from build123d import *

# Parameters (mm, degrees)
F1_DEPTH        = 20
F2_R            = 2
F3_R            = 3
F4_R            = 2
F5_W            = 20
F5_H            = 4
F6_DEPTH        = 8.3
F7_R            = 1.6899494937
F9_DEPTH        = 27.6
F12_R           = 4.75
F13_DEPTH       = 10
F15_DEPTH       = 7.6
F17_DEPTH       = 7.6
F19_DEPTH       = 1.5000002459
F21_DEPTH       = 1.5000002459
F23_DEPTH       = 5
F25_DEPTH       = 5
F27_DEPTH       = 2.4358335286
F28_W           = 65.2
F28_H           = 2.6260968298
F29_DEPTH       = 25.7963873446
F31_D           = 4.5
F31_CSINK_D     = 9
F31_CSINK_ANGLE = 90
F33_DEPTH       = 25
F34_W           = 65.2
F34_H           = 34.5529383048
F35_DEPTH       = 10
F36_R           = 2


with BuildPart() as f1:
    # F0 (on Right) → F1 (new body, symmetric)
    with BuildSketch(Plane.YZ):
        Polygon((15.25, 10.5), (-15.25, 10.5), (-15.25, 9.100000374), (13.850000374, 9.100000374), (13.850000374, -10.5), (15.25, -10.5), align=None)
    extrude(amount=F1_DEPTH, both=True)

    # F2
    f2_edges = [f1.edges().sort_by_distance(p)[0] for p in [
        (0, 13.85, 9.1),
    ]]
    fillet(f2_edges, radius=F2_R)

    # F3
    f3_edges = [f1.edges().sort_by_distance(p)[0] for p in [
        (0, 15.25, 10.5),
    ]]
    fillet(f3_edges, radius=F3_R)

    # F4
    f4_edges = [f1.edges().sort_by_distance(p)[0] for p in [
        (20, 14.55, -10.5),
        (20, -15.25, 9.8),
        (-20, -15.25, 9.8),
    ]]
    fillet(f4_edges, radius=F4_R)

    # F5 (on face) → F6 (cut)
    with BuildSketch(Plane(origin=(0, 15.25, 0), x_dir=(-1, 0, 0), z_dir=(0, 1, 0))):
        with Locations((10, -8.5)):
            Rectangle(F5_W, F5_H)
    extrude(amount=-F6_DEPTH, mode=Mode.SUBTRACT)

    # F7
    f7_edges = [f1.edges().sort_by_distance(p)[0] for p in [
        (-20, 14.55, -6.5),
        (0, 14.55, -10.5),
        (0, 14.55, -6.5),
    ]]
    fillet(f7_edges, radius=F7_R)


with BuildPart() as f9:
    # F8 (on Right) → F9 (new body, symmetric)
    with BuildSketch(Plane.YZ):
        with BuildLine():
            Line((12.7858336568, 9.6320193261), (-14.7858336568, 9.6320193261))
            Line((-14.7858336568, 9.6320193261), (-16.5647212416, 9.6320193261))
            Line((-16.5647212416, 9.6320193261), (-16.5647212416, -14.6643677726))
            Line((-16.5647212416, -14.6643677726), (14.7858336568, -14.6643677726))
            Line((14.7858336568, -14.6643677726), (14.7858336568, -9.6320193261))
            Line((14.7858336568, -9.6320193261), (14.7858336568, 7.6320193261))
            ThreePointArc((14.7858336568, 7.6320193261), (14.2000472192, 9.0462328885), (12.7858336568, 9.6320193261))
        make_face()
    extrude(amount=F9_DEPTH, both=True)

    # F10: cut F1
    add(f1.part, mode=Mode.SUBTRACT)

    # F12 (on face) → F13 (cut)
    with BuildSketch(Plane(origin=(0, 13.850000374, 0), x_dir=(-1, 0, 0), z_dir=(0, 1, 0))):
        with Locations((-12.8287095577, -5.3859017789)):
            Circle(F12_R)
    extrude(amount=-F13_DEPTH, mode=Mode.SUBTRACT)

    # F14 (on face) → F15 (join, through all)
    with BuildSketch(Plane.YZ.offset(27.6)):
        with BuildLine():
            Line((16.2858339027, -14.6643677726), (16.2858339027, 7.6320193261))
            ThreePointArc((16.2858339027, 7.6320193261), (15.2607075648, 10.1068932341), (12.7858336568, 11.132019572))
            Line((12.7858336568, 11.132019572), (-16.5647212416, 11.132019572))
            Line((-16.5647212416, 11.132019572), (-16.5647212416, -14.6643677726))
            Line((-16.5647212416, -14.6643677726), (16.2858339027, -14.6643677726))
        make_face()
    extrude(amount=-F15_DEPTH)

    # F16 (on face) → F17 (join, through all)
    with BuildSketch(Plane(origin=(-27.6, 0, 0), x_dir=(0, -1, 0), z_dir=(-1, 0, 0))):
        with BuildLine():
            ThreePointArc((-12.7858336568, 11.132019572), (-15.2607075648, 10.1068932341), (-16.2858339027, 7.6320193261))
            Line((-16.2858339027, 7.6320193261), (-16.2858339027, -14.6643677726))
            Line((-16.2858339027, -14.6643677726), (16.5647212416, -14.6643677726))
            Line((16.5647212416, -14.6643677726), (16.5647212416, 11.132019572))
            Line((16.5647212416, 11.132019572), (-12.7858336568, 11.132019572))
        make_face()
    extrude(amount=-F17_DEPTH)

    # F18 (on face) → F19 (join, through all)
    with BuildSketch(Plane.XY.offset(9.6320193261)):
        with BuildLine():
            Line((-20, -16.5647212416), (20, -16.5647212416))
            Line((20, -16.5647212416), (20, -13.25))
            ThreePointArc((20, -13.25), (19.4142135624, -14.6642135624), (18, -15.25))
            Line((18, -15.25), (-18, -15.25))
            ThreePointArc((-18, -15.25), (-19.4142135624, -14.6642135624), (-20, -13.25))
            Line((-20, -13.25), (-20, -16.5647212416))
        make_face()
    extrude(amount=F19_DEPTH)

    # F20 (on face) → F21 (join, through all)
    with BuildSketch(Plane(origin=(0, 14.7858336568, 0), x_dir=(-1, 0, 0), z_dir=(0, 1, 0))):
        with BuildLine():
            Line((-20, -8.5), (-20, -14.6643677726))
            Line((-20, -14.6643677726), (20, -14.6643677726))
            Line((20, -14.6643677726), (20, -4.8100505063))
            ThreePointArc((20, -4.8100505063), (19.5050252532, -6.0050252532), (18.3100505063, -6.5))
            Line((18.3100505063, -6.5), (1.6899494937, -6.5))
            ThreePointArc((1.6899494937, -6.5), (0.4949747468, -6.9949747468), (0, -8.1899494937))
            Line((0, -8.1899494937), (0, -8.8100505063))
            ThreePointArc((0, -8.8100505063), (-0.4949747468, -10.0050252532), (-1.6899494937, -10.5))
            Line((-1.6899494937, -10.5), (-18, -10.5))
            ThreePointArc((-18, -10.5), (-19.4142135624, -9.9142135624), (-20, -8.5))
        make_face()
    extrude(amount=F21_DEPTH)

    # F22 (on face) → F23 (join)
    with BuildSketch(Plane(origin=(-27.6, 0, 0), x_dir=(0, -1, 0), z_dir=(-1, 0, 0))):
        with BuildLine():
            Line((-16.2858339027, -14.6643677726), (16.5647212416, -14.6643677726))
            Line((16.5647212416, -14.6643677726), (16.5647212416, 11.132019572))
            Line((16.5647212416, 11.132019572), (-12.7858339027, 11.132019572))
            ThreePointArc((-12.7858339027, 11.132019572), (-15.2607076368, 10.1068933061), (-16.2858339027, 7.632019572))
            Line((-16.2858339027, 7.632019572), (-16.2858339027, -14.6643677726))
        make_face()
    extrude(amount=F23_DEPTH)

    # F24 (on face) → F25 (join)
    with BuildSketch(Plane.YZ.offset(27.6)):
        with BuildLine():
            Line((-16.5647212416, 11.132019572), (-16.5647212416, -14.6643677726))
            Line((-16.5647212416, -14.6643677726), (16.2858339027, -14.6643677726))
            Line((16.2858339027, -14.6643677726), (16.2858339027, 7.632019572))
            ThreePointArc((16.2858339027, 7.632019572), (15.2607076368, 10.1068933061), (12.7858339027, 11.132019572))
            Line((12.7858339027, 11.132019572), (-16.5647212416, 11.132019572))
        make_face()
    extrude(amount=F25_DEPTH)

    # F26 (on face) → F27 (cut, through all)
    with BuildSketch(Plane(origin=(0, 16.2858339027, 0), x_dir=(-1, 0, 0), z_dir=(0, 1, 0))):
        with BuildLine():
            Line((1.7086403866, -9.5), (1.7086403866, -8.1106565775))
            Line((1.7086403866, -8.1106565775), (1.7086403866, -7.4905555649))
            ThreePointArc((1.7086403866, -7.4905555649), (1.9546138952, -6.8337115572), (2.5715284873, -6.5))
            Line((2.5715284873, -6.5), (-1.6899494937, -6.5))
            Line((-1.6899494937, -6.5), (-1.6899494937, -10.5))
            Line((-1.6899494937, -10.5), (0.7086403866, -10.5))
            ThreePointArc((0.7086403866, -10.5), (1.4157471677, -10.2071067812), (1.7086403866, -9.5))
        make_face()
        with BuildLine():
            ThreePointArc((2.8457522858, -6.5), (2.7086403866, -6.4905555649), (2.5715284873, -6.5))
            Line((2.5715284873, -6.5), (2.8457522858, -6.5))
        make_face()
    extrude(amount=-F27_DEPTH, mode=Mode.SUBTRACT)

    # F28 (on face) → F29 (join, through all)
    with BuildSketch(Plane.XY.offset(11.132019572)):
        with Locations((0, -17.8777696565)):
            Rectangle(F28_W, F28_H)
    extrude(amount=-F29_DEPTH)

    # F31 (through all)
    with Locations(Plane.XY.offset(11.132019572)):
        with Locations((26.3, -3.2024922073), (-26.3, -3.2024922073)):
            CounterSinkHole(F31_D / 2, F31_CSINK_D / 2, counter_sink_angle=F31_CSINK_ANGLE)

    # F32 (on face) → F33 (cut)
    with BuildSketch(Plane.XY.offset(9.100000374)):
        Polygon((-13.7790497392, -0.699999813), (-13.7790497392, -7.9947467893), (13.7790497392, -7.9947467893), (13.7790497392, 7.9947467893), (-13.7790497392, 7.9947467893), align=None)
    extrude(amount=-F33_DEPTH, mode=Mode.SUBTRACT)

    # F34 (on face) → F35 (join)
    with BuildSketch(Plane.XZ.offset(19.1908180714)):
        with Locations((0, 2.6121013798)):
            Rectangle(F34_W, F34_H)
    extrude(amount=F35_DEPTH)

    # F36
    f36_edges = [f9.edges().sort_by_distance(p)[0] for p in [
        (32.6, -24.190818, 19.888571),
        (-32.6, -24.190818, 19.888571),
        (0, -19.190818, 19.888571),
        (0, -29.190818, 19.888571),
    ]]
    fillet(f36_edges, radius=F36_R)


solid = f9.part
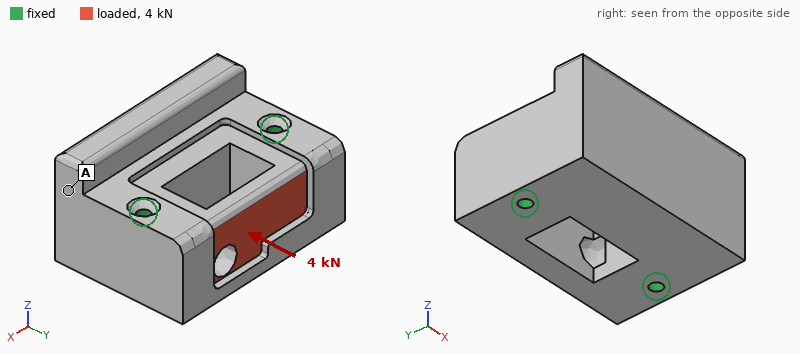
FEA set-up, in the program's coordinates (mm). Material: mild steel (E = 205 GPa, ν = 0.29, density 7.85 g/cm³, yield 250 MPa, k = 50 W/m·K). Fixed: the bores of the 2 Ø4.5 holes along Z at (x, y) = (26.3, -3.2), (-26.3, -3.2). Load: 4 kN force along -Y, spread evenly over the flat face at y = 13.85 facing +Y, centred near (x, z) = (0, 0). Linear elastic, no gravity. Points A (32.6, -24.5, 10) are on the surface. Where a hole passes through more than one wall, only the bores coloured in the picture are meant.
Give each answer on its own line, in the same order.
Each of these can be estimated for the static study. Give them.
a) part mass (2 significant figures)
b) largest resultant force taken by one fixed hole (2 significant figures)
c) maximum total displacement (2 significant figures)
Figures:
520 g
2.1 kN
8.7 µm
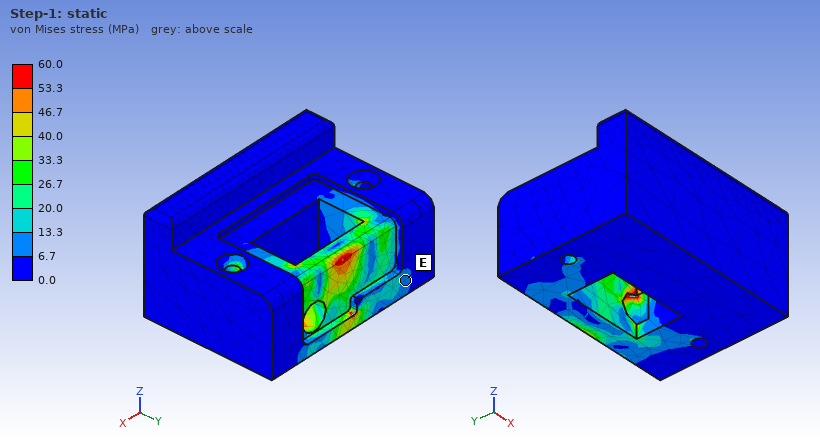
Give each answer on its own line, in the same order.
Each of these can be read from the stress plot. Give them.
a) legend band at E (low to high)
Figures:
6.7 to 13.3 MPa
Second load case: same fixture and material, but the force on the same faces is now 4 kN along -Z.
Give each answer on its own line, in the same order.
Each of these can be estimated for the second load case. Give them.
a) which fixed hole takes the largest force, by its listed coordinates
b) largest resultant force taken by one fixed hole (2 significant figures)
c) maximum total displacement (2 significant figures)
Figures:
(-26.3, -3.2)
2.2 kN
7.8 µm
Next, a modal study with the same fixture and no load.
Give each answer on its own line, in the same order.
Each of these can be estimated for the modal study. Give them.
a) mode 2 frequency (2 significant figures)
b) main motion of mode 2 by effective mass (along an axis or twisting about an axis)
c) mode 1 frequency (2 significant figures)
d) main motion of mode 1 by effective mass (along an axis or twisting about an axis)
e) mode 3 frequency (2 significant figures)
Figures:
16 kHz
along X
11 kHz
along Z
18 kHz
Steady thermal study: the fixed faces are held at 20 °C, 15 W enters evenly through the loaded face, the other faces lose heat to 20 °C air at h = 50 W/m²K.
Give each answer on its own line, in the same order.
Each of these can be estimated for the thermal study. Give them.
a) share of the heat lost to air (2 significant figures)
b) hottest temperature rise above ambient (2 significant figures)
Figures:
11 %
16 K
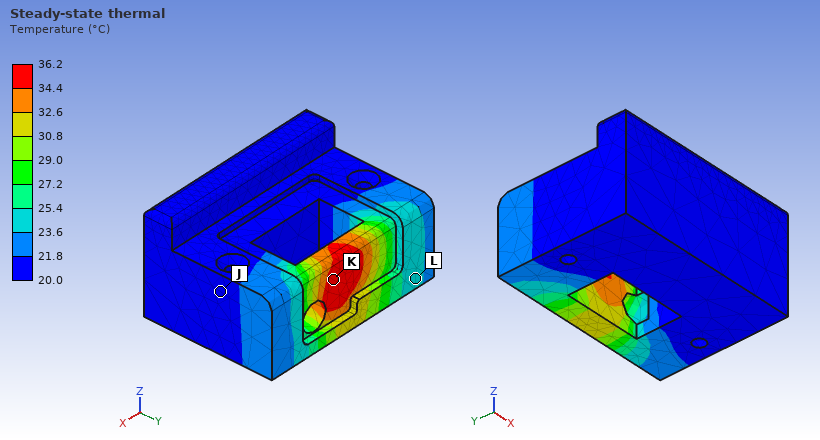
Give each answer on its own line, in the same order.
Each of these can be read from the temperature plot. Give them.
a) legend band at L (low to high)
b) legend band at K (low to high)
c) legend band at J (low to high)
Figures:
23.6 to 25.4 °C
34.4 to 36.2 °C
20.0 to 21.8 °C
